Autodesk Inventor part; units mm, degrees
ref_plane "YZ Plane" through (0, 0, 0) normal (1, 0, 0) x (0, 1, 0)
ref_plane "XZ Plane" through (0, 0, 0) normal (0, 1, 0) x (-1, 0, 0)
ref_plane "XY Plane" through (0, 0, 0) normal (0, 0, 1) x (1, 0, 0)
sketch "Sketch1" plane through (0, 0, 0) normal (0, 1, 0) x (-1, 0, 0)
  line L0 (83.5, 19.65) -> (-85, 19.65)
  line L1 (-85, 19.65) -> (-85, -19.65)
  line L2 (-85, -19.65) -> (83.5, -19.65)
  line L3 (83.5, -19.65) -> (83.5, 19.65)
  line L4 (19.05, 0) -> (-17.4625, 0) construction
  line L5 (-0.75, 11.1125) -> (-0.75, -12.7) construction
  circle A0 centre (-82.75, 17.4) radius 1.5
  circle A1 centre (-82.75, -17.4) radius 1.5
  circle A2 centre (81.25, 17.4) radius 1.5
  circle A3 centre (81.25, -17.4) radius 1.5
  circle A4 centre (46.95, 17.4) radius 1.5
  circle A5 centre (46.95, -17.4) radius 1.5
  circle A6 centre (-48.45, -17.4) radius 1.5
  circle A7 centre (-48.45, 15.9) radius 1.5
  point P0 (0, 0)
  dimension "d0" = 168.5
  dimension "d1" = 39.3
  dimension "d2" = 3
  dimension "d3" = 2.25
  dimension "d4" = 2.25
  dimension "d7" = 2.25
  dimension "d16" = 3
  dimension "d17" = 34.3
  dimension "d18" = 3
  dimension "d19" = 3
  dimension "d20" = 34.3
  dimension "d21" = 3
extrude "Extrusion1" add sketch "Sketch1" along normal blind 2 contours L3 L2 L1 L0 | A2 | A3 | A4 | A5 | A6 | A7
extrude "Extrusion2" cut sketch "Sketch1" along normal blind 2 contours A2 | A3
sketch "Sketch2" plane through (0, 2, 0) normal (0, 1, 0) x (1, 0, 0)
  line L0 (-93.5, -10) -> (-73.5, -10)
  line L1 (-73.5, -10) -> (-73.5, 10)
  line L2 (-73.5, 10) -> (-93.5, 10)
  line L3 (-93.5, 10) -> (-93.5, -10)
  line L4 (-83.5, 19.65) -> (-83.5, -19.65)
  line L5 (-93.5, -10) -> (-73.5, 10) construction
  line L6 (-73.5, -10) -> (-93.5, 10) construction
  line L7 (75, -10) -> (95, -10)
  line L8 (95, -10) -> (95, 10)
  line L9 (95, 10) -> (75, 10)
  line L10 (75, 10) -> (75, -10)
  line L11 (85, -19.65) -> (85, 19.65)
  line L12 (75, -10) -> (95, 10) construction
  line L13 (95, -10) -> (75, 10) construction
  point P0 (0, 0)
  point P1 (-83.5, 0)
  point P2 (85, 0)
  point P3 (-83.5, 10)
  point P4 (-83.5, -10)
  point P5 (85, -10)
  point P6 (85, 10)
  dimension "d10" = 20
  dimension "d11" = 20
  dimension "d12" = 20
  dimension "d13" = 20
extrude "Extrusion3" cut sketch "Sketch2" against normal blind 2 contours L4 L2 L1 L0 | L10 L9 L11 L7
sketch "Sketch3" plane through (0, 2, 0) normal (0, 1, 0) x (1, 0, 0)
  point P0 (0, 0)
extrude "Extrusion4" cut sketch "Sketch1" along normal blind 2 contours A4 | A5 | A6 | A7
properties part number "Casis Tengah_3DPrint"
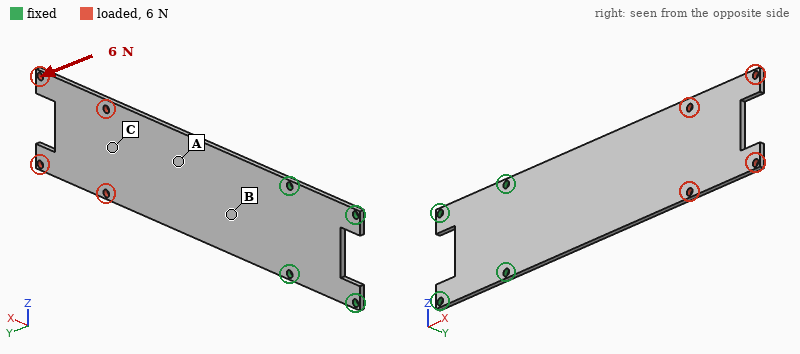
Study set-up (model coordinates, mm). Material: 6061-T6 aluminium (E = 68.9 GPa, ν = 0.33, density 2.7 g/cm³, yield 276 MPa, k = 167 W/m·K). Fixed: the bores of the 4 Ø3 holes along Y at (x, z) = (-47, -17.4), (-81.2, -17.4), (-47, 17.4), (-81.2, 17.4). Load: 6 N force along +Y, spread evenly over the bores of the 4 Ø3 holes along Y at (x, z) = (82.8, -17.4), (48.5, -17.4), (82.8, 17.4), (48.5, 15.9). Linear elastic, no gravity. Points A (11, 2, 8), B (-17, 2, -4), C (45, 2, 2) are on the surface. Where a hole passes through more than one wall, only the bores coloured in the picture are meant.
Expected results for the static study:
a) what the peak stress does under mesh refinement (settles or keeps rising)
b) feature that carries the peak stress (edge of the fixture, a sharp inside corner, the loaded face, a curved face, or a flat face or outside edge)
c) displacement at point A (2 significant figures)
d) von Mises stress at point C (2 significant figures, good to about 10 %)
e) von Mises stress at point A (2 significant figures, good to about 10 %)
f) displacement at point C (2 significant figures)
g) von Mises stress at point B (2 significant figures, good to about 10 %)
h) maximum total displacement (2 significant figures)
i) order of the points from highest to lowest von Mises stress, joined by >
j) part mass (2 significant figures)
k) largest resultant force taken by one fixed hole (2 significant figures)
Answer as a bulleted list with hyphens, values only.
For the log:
- keeps rising
- edge of the fixture
- 0.55 mm
- 4.9 MPa
- 13 MPa
- 1.2 mm
- 19 MPa
- 2.1 mm
- B > A > C
- 33 g
- 6.5 N
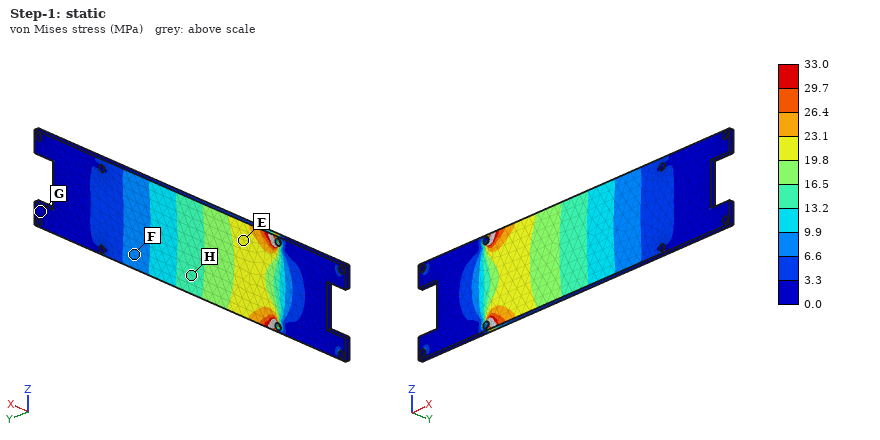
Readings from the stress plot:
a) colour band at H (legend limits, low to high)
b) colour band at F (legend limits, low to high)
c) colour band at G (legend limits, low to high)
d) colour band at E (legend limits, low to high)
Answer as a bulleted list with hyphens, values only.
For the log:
- 13.2 to 16.5 MPa
- 6.6 to 9.9 MPa
- 0.0 to 3.3 MPa
- 19.8 to 23.1 MPa
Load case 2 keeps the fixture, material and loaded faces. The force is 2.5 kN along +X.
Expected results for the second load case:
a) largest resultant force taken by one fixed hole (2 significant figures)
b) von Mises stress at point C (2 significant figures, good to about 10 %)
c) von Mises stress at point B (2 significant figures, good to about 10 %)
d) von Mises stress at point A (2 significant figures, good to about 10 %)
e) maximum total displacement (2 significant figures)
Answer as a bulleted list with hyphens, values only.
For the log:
- 1.1 kN
- 21 MPa
- 31 MPa
- 31 MPa
- 91 µm
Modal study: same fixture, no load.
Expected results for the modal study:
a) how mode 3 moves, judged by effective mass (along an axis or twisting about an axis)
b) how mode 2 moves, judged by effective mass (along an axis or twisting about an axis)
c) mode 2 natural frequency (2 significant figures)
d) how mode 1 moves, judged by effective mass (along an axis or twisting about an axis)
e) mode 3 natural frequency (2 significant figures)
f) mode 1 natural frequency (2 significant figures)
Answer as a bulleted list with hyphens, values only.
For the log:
- twisting about X
- along Y
- 620 Hz
- along Y
- 650 Hz
- 100 Hz
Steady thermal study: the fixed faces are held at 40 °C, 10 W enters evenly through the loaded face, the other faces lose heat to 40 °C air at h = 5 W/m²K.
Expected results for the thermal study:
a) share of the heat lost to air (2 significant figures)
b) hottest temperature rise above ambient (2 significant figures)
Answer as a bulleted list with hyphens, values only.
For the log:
- 22 %
- 84 K
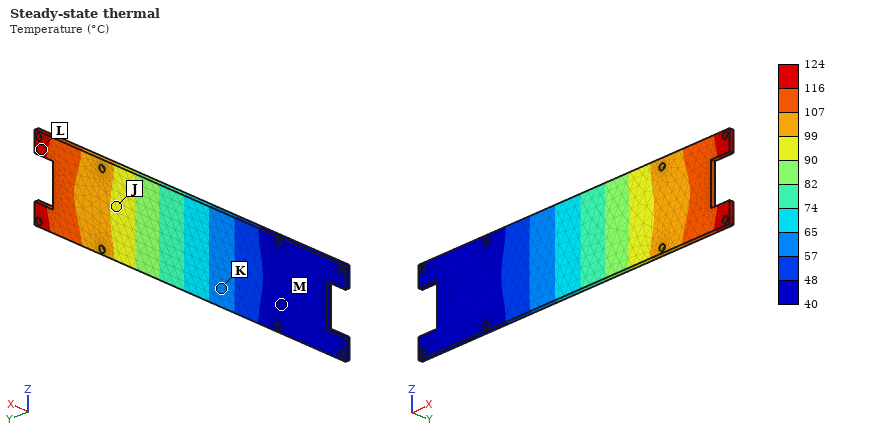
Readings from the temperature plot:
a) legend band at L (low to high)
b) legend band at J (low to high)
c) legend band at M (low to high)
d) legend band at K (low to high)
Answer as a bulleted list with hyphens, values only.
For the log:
- 116 to 124 °C
- 90 to 99 °C
- 40 to 48 °C
- 57 to 65 °C
